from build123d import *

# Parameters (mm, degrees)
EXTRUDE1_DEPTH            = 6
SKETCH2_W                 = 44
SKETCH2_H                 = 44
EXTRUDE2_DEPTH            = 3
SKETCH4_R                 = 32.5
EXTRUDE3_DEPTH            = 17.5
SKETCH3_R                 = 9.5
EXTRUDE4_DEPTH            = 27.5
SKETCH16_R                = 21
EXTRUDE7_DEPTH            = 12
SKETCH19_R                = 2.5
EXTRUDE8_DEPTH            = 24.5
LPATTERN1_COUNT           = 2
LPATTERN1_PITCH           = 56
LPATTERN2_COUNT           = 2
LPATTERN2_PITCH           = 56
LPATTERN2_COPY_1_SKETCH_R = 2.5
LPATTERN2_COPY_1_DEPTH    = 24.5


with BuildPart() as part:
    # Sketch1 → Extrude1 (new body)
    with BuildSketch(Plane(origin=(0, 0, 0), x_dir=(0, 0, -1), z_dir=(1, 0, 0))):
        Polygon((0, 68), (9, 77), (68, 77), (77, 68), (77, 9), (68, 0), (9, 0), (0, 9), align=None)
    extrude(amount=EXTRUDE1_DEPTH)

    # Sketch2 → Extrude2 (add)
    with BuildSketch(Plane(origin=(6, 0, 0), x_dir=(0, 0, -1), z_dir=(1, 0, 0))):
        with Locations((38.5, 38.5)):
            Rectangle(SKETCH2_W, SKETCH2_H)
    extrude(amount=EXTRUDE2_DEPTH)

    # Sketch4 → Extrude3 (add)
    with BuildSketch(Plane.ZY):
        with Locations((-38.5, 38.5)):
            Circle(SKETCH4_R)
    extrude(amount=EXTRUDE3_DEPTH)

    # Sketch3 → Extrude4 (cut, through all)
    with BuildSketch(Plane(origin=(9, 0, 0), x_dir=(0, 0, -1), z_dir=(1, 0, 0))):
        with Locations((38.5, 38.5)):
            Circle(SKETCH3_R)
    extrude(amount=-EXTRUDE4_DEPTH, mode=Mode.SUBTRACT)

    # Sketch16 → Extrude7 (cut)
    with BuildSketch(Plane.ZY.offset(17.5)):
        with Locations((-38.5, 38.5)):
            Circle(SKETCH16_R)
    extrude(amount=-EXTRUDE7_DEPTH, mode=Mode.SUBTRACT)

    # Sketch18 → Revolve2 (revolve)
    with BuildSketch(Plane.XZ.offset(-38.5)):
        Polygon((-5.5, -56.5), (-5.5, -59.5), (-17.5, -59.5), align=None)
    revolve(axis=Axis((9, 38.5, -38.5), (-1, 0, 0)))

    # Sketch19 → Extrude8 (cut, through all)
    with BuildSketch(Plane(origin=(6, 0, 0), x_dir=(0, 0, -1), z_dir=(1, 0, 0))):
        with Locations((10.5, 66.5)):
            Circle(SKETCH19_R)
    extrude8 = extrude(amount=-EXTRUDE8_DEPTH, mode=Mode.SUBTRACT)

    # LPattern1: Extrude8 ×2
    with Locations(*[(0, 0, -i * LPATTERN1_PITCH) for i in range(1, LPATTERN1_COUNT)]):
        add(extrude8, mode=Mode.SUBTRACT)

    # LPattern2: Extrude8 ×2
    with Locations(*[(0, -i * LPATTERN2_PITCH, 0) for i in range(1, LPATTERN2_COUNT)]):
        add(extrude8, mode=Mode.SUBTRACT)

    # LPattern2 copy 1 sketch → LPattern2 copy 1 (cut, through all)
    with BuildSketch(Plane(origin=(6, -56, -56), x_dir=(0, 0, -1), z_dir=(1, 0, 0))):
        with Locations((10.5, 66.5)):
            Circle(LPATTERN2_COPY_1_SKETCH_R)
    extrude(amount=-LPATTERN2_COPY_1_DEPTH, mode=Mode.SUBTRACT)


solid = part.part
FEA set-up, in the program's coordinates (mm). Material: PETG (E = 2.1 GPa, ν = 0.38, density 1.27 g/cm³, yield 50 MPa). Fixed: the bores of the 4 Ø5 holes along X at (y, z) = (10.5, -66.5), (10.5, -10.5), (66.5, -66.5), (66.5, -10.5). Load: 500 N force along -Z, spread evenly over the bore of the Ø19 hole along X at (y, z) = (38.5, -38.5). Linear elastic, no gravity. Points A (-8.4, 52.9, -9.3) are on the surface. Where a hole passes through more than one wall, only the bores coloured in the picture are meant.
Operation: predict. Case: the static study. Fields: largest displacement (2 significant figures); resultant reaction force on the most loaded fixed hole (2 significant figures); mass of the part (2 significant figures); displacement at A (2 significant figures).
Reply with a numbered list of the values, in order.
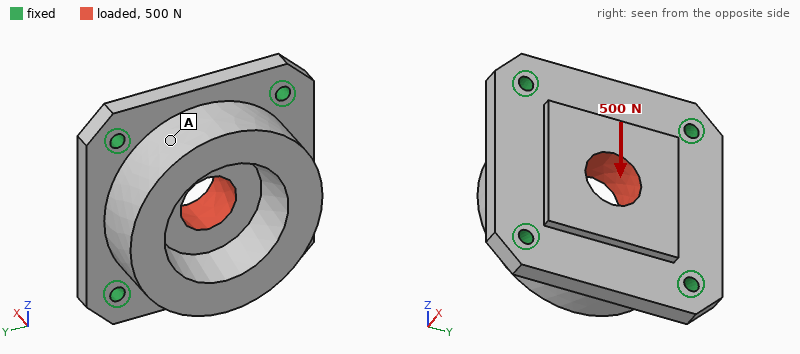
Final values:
1. 17 µm
2. 130 N
3. 100 g
4. 10 µm
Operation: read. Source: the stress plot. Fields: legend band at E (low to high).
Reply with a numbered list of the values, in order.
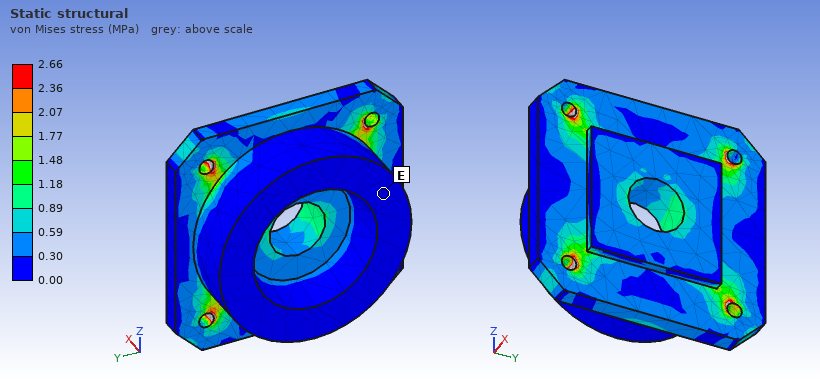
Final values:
1. 0.00 to 0.30 MPa
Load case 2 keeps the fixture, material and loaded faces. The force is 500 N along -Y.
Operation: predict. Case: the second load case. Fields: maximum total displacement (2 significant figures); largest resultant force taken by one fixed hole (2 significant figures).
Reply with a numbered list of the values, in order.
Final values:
1. 17 µm
2. 130 N
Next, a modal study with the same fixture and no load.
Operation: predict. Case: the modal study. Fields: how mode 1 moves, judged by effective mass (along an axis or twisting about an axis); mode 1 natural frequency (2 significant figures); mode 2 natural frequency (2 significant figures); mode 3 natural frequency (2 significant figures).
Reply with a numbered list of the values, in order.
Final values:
1. along X
2. 2100 Hz
3. 2600 Hz
4. 2600 Hz
